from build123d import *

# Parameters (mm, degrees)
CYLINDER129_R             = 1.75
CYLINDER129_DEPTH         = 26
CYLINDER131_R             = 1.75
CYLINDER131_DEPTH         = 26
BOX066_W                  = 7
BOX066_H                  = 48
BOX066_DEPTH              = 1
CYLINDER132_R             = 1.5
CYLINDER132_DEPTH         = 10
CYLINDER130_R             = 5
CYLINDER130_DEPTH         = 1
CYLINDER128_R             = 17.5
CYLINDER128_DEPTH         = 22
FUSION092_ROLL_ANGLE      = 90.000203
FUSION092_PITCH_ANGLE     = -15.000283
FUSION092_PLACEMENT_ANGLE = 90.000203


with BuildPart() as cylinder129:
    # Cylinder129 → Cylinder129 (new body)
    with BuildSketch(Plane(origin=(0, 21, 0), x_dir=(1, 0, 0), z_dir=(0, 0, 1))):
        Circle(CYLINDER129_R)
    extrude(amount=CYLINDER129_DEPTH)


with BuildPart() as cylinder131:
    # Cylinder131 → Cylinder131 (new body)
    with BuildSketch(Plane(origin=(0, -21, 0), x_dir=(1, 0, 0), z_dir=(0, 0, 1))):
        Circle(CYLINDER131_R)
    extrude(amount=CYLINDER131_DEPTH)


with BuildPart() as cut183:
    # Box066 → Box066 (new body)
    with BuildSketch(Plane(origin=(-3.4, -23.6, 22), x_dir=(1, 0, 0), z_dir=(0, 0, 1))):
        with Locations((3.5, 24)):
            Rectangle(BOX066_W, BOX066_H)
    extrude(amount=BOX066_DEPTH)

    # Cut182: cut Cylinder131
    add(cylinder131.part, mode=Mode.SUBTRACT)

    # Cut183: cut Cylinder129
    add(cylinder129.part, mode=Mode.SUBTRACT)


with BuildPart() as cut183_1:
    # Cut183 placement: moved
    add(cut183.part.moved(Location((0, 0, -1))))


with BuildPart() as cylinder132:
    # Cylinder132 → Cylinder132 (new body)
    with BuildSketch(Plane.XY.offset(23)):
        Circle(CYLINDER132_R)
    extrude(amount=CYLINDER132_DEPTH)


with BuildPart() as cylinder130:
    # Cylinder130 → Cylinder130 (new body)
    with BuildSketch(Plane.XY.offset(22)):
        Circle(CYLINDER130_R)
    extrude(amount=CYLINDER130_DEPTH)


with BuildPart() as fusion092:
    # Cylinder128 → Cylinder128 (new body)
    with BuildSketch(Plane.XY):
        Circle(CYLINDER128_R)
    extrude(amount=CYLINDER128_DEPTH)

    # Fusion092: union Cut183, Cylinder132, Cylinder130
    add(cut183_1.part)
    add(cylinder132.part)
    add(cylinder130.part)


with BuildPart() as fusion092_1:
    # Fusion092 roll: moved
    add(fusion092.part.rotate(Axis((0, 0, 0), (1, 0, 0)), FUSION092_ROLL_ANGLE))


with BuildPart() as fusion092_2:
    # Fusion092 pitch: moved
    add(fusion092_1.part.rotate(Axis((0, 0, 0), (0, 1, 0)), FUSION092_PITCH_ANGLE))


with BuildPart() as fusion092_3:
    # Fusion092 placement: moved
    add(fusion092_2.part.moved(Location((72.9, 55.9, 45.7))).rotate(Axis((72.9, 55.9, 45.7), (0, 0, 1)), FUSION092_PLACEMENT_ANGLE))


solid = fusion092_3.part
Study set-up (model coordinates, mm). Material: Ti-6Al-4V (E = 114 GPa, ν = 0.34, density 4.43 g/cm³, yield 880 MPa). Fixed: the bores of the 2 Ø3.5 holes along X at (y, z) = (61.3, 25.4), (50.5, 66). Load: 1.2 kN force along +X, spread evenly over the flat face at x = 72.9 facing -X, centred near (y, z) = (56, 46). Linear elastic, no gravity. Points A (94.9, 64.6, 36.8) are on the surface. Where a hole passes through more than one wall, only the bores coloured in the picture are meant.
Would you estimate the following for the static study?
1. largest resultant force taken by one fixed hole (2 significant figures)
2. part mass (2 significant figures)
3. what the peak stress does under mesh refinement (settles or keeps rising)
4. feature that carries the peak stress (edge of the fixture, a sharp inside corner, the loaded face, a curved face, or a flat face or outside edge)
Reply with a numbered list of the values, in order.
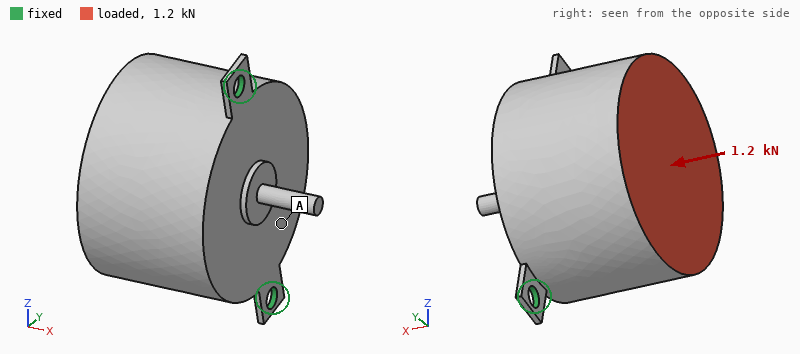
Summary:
1. 690 N
2. 95 g
3. keeps rising
4. edge of the fixture
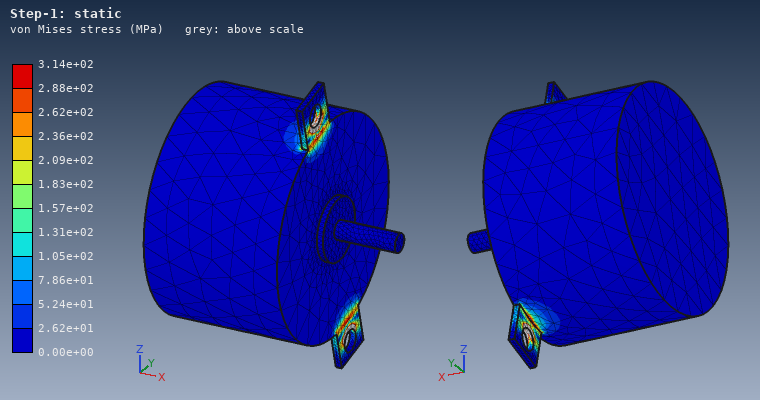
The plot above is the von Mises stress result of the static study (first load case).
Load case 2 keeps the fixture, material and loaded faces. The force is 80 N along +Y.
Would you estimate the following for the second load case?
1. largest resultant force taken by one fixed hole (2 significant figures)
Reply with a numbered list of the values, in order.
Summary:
1. 42 N
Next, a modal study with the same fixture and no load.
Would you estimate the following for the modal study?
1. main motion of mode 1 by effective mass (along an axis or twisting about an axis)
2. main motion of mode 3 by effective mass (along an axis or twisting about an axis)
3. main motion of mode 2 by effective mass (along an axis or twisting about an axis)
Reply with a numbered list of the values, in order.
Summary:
1. along Y
2. along Z
3. along X
